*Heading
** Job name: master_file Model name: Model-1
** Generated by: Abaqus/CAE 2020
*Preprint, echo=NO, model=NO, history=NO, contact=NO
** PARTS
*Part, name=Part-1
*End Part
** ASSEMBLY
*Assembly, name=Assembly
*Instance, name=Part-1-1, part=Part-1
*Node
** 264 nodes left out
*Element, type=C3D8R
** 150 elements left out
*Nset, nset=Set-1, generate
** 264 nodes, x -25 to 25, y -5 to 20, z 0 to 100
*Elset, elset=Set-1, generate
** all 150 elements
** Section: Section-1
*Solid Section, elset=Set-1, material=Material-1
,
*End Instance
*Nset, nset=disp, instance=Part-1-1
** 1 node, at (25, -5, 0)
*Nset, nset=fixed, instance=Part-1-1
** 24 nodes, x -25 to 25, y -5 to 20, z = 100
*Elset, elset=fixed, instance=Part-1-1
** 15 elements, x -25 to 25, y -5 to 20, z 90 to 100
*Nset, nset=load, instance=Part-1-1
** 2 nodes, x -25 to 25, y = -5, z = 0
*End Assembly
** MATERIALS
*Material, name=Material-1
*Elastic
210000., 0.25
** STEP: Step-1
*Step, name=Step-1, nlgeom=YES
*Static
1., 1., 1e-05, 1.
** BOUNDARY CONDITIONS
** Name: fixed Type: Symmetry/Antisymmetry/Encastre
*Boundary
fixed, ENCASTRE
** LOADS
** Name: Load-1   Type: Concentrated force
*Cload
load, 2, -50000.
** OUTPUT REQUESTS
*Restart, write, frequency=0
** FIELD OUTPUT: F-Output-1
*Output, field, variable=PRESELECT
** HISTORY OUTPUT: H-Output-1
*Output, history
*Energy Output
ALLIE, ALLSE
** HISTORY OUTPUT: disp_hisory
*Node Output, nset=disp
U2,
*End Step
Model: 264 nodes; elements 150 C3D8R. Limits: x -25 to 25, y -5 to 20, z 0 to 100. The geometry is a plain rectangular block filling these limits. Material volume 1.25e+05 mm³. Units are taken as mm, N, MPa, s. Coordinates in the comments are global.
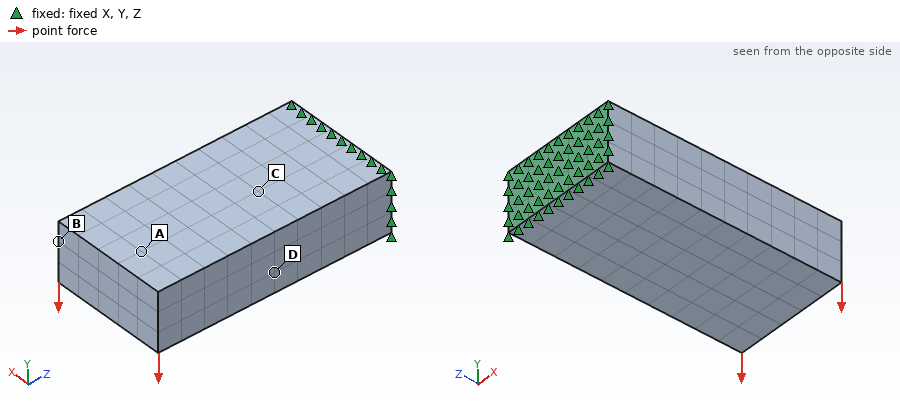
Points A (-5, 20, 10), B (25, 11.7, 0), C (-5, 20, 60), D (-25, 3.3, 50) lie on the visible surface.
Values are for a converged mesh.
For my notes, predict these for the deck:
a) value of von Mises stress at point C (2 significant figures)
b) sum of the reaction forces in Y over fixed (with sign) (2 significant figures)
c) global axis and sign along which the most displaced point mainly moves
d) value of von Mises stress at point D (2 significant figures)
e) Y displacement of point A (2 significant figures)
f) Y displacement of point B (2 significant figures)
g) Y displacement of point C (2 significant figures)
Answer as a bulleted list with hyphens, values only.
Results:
- 1100 MPa
- 1.0e+05 N
- -Y
- 410 MPa
- -2.1 mm
- -2.5 mm
- -0.55 mm
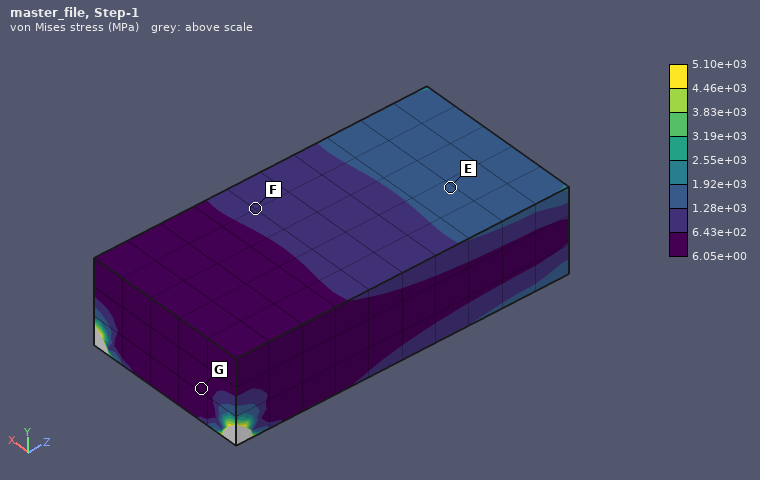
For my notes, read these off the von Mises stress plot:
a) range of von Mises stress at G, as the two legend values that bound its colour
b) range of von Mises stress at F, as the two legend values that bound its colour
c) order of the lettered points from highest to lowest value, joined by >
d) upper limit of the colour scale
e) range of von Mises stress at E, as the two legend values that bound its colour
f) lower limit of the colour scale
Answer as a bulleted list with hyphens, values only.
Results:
- 6.05e+00 to 6.43e+02 MPa
- 6.43e+02 to 1.28e+03 MPa
- E > F > G
- 5.10e+03 MPa
- 1.28e+03 to 1.92e+03 MPa
- 6.05e+00 MPa
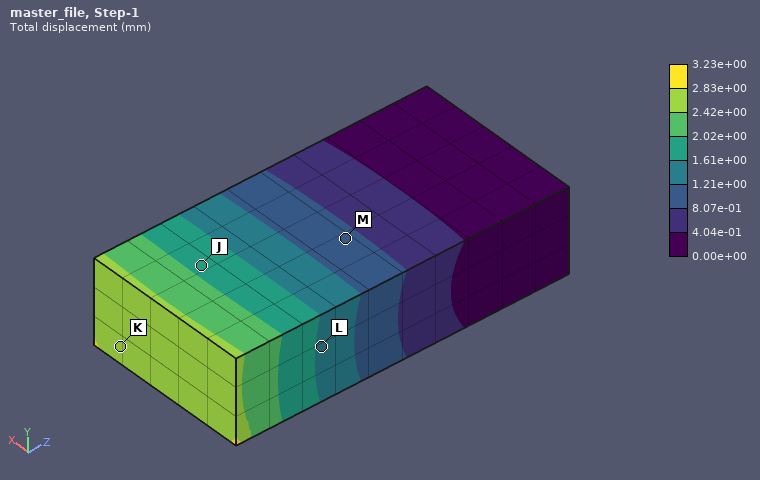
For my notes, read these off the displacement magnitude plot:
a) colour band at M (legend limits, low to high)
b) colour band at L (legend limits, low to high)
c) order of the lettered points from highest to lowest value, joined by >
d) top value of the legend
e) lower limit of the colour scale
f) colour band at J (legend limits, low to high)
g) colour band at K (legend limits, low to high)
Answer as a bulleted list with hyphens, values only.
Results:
- 8.07e-01 to 1.21e+00 mm
- 1.21e+00 to 1.61e+00 mm
- K > J > L > M
- 3.23e+00 mm
- 0.00e+00 mm
- 1.61e+00 to 2.02e+00 mm
- 2.42e+00 to 2.83e+00 mm
